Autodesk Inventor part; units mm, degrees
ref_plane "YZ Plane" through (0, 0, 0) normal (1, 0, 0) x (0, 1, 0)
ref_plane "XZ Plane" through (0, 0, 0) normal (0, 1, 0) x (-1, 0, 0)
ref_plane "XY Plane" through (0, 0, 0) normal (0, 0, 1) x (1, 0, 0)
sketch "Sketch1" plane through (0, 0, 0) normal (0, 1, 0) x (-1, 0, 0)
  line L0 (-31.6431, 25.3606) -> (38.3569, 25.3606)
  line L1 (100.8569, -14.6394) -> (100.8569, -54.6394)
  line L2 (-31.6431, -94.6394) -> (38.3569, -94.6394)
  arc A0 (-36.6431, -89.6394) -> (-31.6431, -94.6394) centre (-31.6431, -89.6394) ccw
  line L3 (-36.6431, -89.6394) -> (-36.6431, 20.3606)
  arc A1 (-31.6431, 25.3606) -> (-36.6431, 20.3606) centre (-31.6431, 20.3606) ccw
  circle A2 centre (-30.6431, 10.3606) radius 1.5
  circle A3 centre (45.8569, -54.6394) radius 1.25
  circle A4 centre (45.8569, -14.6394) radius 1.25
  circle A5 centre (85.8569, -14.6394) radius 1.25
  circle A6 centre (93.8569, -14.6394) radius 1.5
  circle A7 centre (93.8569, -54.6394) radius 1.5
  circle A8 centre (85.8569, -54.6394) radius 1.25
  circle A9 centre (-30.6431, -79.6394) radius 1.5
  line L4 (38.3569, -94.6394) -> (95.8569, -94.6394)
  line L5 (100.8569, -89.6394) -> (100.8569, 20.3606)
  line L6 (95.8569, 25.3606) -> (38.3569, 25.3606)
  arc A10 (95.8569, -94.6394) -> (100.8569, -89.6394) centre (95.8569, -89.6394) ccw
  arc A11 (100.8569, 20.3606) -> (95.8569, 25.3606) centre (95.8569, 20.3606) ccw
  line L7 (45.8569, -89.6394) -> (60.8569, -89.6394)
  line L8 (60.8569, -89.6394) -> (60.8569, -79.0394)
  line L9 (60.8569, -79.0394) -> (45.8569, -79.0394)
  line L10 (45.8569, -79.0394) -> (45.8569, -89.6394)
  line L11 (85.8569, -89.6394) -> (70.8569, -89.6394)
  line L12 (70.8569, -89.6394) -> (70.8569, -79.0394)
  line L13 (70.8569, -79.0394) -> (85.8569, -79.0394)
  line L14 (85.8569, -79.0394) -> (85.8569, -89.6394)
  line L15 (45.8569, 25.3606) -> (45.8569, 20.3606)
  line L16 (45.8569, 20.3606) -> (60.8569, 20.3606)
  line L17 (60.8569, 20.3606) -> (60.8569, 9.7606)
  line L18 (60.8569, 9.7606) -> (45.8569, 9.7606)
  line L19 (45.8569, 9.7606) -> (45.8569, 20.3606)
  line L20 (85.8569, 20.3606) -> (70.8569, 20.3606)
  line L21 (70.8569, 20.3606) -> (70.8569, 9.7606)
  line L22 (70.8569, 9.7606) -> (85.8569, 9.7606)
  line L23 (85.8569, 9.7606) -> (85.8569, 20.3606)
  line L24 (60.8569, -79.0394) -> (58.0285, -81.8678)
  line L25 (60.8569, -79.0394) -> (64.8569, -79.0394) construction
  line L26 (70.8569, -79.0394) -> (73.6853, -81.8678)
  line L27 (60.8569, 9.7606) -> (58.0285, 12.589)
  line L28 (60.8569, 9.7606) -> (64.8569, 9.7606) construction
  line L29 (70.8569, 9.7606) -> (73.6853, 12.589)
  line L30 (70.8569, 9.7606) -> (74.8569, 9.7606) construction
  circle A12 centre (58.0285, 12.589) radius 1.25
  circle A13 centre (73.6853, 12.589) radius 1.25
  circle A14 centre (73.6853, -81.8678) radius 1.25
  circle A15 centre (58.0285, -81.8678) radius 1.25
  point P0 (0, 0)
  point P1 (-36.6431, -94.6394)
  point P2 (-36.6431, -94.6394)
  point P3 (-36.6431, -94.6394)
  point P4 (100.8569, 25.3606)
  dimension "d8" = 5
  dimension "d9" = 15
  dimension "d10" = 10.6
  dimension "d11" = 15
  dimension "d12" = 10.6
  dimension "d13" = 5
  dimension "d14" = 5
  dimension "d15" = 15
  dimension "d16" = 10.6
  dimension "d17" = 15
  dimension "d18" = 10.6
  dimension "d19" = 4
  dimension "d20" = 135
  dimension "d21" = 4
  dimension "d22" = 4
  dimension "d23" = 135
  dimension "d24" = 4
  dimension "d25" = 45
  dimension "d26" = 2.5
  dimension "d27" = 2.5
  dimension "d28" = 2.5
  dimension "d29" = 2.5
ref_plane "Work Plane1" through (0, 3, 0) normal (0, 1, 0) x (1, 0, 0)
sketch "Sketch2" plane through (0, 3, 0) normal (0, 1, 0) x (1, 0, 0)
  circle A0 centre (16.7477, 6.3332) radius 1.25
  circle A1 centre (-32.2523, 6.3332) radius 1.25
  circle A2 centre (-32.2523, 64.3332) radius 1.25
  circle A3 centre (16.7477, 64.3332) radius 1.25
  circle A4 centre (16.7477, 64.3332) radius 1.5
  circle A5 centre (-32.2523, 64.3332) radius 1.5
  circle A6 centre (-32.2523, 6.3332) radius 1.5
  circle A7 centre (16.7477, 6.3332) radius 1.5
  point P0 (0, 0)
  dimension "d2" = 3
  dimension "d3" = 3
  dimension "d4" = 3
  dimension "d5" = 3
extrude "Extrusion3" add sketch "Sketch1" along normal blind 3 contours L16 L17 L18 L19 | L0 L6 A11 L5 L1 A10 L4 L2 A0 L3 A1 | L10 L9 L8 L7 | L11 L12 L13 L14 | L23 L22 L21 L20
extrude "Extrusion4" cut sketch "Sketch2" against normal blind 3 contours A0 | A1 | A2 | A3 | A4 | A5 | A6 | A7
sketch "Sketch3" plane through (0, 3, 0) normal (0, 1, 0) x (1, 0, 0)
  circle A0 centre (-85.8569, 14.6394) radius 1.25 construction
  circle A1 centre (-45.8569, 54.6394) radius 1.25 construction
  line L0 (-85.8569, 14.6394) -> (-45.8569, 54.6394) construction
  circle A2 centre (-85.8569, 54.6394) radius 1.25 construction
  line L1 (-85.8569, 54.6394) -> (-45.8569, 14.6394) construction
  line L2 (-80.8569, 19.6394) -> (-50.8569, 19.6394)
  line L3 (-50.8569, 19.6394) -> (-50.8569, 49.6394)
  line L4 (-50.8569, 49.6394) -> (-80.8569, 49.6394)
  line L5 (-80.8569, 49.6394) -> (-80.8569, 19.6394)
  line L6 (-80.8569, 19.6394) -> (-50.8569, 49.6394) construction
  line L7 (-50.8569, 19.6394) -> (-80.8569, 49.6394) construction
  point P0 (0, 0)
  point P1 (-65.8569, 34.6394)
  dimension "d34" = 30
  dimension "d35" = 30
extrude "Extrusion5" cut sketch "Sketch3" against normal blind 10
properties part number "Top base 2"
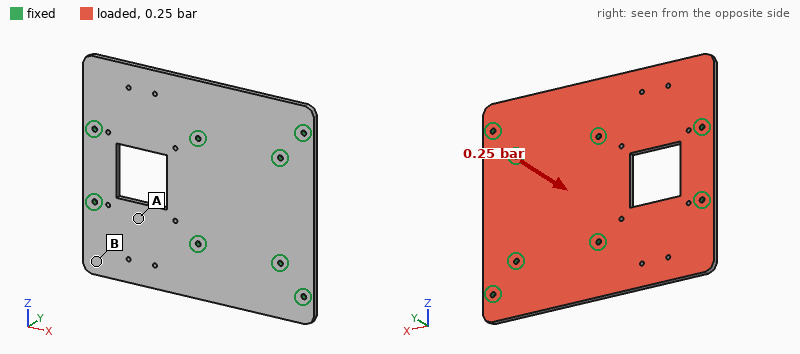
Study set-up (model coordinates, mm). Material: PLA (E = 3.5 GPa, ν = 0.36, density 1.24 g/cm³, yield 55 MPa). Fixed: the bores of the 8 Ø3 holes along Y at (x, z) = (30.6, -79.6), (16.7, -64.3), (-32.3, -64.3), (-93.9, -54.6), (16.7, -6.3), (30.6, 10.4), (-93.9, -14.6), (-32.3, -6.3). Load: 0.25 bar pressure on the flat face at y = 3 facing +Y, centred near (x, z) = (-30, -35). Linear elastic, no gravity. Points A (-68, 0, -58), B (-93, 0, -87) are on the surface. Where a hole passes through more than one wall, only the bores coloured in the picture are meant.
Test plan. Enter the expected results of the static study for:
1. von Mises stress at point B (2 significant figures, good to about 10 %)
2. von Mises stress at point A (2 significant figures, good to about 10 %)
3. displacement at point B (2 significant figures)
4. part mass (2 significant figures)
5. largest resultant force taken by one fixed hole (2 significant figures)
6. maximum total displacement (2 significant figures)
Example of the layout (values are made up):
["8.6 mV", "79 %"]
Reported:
["1.4 MPa", "3.6 MPa", "0.84 mm", "58 g", "87 N", "1.1 mm"]
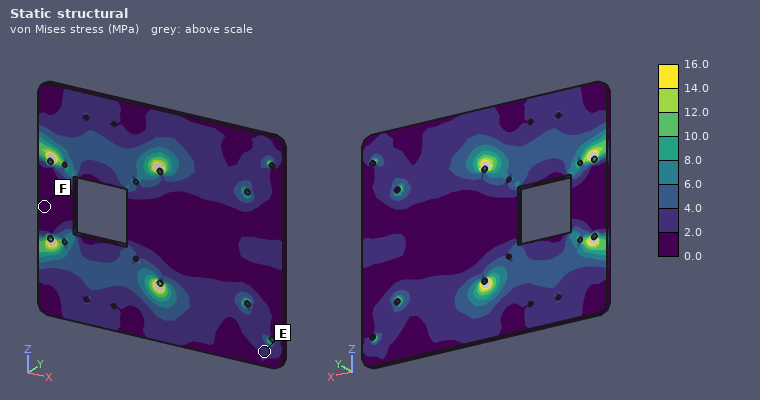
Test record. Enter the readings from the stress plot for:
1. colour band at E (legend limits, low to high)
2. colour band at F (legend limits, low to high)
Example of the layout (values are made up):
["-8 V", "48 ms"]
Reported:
["2.0 to 4.0 MPa", "0.0 to 2.0 MPa"]
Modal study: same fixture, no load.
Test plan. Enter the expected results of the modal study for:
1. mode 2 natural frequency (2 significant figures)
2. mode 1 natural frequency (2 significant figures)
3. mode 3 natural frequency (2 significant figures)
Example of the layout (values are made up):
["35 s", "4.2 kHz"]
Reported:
["520 Hz", "500 Hz", "880 Hz"]
